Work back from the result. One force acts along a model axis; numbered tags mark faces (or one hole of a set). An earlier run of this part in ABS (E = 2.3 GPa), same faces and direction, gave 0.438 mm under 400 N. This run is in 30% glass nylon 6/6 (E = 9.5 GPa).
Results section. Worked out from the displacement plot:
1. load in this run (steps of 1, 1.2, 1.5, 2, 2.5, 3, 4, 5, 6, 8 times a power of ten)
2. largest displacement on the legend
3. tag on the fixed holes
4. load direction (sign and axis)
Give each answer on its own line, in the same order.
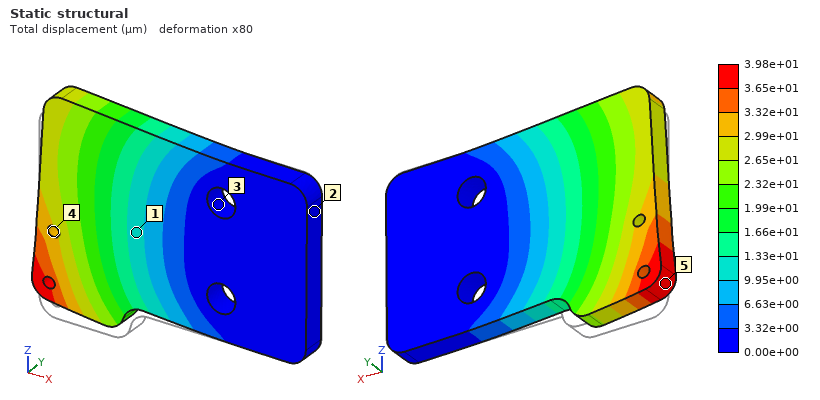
150 N
3.98e+01 µm
3
+Z
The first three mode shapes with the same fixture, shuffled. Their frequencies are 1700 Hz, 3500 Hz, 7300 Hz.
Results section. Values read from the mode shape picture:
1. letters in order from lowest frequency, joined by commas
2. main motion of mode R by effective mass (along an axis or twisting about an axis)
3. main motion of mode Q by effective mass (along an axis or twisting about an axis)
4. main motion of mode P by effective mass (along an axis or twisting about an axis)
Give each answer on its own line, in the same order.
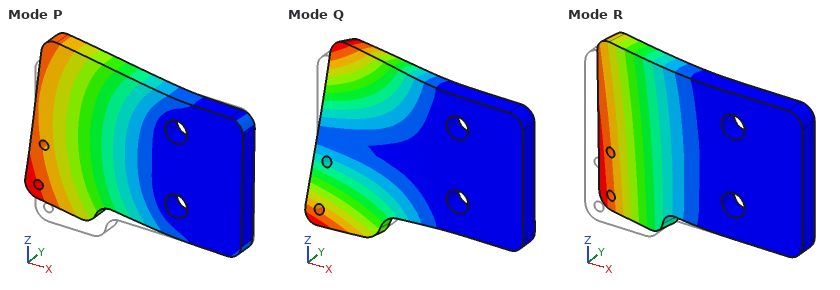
R, Q, P
along Y
twisting about X
along Z
